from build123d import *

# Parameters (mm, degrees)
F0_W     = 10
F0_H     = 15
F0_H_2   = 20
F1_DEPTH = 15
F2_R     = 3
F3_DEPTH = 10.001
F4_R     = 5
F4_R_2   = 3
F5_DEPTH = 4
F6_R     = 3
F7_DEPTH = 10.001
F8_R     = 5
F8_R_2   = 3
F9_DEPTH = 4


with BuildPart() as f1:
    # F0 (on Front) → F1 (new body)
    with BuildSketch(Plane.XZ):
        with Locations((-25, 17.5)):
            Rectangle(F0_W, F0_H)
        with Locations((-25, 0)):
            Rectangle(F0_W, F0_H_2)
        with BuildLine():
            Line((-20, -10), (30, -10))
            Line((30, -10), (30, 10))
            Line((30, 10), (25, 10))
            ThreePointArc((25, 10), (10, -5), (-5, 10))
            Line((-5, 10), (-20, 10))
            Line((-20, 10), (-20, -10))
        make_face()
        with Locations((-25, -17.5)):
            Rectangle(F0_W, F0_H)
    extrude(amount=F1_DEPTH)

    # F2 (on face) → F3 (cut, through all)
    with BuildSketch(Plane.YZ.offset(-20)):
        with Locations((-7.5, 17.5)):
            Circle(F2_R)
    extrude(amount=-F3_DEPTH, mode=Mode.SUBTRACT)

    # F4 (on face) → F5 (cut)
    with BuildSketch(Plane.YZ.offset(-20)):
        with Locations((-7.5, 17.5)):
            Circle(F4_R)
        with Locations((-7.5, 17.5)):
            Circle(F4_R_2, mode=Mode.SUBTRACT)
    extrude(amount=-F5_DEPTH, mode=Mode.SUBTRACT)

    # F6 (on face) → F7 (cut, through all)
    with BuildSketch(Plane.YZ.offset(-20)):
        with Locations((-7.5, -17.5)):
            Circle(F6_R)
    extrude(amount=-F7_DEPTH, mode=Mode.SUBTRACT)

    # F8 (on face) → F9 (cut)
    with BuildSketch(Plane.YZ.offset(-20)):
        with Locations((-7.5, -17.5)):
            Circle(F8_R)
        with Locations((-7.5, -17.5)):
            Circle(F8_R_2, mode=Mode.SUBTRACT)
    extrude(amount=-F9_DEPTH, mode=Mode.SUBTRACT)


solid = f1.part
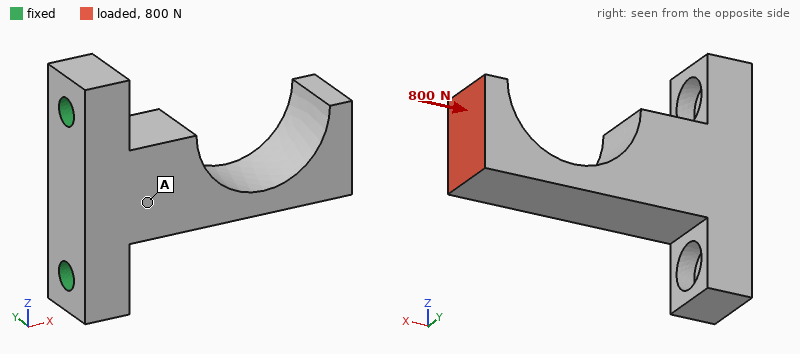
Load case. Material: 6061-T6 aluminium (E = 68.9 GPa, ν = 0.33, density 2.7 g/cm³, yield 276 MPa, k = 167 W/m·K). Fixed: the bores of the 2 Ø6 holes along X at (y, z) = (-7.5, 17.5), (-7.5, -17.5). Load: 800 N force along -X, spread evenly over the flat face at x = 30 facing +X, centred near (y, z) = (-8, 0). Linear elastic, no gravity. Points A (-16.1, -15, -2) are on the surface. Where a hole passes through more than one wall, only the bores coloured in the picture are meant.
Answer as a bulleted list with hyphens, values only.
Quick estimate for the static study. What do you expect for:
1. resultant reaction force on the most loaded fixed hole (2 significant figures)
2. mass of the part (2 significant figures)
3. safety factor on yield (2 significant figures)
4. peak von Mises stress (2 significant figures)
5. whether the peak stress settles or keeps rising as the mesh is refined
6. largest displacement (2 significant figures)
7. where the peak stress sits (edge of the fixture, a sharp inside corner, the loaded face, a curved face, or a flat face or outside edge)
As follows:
- 450 N
- 44 g
- 2.6
- 110 MPa
- settles
- 0.21 mm
- a curved face
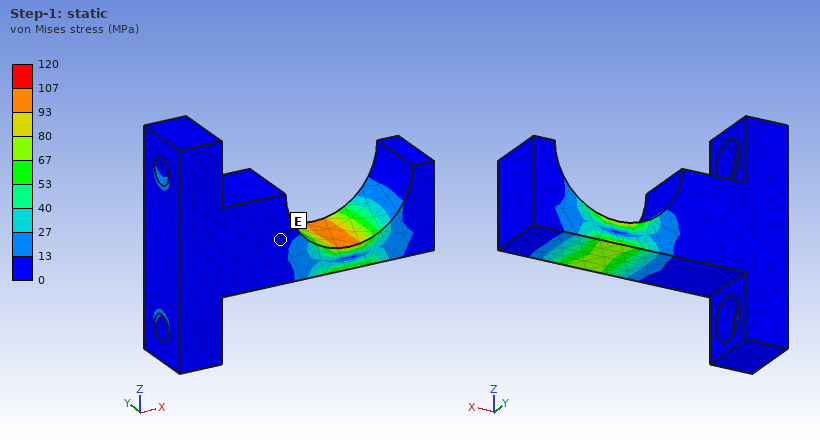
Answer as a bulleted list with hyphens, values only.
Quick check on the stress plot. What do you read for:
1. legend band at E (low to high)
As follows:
- 0 to 13 MPa
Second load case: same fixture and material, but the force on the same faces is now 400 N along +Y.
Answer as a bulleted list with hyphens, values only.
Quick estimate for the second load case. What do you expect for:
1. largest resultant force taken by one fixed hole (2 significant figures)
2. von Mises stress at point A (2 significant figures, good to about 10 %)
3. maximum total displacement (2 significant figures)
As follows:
- 200 N
- 21 MPa
- 0.26 mm
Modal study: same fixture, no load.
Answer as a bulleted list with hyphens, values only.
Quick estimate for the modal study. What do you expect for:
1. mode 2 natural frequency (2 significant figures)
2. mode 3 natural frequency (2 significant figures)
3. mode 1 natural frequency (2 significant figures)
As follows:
- 2500 Hz
- 7400 Hz
- 2500 Hz
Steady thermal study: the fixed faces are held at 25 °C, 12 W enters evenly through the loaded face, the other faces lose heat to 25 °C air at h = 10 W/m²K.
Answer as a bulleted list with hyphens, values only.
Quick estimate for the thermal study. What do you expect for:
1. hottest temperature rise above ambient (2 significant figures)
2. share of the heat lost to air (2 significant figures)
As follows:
- 32 K
- 4.1 %
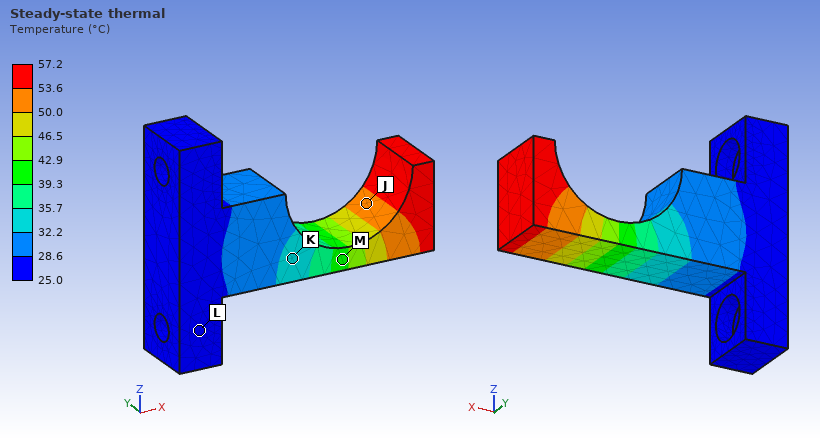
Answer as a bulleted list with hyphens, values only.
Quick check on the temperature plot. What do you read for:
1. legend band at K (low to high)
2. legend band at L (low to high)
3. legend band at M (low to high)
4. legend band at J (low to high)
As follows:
- 32.2 to 35.7 °C
- 25.0 to 28.6 °C
- 39.3 to 42.9 °C
- 50.0 to 53.6 °C
